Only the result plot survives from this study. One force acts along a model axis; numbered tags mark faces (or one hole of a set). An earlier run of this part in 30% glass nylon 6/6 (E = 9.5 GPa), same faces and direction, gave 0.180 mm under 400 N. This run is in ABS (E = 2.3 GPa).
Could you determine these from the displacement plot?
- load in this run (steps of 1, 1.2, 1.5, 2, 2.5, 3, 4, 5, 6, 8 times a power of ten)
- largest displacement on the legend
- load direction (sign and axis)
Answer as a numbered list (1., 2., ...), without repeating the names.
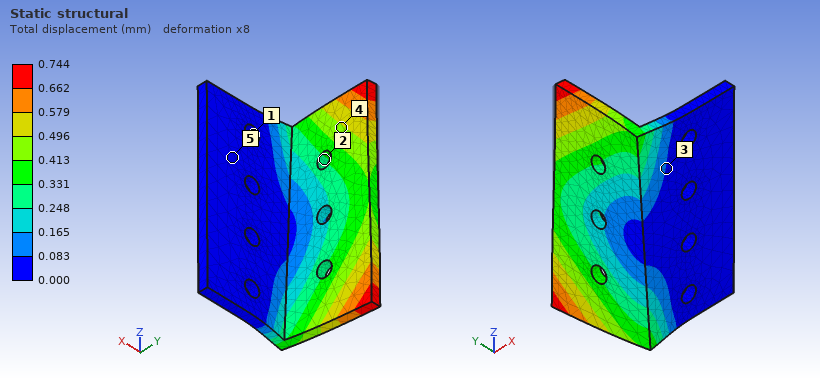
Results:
1. 400 N
2. 0.744 mm
3. -Z
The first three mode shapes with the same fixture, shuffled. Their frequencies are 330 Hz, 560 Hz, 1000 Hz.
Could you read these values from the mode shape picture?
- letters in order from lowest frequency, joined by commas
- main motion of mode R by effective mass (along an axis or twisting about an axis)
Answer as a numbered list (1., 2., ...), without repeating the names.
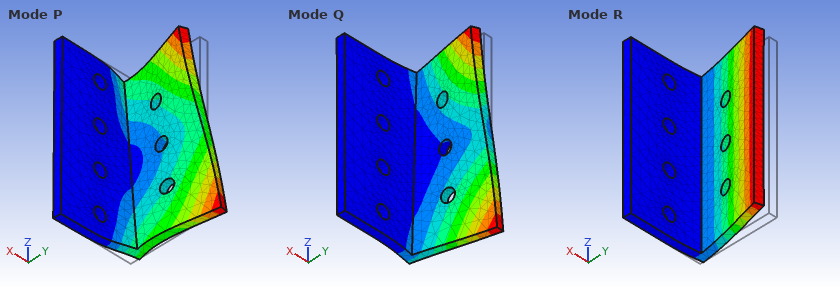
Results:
1. R, Q, P
2. along X
